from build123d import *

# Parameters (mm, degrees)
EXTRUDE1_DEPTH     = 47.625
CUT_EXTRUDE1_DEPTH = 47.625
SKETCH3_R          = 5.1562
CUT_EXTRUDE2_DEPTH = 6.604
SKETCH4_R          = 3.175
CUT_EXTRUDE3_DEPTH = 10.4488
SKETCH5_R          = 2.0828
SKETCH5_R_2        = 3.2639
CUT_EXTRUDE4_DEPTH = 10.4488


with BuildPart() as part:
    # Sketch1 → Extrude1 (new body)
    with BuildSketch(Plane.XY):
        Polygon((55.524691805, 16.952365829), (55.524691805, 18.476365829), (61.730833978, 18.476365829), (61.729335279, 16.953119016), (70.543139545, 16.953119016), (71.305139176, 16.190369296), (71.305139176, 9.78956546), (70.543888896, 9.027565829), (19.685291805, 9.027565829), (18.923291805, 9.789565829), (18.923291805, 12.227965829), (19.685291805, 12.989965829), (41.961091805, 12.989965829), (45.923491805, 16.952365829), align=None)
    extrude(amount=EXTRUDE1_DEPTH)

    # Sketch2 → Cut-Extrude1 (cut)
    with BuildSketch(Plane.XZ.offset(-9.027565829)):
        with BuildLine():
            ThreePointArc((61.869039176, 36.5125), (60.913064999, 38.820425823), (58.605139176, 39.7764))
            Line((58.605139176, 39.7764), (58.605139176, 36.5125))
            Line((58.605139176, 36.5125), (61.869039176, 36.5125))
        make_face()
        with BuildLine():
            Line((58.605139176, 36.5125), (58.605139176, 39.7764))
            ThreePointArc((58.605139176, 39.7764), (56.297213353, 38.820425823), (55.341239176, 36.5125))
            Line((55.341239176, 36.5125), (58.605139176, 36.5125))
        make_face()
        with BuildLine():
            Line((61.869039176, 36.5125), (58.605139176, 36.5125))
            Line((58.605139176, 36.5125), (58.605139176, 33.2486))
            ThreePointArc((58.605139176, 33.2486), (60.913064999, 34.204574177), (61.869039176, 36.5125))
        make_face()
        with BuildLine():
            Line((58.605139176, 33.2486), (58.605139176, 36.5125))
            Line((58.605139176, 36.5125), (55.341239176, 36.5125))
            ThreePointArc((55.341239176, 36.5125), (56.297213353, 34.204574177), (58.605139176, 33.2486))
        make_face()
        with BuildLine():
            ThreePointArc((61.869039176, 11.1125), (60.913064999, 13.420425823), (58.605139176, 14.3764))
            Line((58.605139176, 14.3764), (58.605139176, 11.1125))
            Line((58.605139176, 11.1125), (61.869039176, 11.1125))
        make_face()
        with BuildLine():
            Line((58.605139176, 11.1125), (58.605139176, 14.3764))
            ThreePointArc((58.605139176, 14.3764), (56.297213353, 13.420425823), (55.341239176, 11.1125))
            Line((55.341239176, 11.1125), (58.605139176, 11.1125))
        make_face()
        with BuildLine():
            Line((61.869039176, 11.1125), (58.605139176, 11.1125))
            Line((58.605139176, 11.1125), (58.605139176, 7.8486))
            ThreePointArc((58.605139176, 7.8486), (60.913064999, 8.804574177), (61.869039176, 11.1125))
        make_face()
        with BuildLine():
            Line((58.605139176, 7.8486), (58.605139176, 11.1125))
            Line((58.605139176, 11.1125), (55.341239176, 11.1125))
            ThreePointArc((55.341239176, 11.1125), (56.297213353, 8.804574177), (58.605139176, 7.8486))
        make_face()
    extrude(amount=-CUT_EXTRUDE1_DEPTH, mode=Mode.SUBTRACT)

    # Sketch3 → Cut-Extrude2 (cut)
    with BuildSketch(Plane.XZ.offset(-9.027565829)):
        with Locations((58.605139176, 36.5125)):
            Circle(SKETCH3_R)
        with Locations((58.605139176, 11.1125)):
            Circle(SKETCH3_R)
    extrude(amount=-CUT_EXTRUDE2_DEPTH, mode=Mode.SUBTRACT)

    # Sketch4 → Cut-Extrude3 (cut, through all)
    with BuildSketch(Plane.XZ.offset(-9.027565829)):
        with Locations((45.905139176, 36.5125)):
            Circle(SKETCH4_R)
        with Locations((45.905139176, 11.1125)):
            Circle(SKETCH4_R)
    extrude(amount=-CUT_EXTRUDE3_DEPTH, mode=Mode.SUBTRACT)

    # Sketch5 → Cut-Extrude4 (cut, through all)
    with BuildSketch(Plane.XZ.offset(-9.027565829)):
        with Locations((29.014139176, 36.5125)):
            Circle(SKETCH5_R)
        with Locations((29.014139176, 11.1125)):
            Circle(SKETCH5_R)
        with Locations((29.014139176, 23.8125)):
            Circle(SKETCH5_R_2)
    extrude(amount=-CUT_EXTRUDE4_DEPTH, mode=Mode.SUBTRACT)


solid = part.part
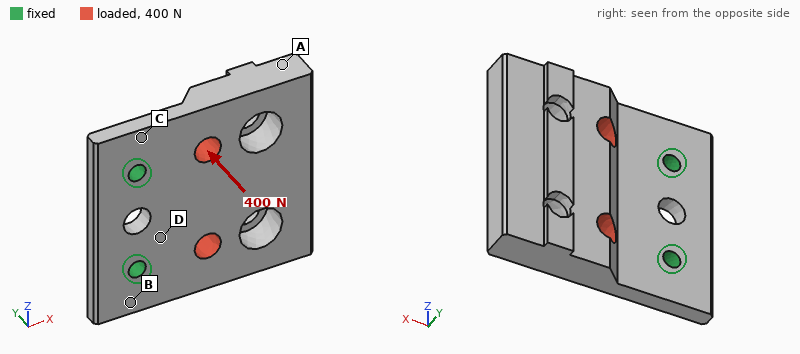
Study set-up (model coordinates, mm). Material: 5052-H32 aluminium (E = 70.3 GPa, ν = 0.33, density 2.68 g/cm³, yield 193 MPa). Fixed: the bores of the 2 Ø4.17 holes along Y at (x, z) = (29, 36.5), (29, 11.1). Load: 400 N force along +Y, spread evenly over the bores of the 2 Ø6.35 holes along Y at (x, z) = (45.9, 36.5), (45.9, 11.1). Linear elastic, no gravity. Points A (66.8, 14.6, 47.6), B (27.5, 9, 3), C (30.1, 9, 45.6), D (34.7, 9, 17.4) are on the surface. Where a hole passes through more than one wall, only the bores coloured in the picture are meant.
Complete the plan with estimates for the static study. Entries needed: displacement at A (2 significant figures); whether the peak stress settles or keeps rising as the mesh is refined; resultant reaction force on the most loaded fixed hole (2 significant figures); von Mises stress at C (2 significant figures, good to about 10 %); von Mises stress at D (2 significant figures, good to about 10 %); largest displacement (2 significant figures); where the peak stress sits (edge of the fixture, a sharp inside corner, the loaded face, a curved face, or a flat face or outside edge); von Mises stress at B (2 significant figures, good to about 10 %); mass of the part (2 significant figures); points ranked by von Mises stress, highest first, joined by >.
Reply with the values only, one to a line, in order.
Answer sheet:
0.12 mm
keeps rising
200 N
24 MPa
32 MPa
0.13 mm
edge of the fixture
15 MPa
36 g
D > C > B > A
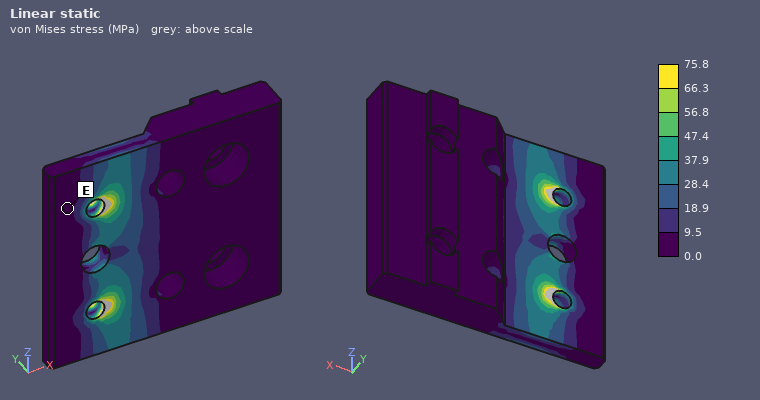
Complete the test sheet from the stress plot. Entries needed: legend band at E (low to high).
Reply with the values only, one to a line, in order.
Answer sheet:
0.0 to 9.5 MPa
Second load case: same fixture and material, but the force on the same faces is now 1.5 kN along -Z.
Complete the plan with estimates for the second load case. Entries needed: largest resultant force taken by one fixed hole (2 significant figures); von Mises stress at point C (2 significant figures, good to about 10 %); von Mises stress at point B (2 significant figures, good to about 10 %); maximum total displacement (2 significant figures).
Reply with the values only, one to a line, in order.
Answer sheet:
1.2 kN
12 MPa
12 MPa
19 µm
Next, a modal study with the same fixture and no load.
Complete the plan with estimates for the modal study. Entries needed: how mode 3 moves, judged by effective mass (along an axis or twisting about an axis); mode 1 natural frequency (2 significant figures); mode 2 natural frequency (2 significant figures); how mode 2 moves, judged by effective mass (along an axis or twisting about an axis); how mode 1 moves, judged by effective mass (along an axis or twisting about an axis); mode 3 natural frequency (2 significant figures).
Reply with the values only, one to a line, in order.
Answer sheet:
along Z
1400 Hz
4400 Hz
twisting about X
along Y
8000 Hz
